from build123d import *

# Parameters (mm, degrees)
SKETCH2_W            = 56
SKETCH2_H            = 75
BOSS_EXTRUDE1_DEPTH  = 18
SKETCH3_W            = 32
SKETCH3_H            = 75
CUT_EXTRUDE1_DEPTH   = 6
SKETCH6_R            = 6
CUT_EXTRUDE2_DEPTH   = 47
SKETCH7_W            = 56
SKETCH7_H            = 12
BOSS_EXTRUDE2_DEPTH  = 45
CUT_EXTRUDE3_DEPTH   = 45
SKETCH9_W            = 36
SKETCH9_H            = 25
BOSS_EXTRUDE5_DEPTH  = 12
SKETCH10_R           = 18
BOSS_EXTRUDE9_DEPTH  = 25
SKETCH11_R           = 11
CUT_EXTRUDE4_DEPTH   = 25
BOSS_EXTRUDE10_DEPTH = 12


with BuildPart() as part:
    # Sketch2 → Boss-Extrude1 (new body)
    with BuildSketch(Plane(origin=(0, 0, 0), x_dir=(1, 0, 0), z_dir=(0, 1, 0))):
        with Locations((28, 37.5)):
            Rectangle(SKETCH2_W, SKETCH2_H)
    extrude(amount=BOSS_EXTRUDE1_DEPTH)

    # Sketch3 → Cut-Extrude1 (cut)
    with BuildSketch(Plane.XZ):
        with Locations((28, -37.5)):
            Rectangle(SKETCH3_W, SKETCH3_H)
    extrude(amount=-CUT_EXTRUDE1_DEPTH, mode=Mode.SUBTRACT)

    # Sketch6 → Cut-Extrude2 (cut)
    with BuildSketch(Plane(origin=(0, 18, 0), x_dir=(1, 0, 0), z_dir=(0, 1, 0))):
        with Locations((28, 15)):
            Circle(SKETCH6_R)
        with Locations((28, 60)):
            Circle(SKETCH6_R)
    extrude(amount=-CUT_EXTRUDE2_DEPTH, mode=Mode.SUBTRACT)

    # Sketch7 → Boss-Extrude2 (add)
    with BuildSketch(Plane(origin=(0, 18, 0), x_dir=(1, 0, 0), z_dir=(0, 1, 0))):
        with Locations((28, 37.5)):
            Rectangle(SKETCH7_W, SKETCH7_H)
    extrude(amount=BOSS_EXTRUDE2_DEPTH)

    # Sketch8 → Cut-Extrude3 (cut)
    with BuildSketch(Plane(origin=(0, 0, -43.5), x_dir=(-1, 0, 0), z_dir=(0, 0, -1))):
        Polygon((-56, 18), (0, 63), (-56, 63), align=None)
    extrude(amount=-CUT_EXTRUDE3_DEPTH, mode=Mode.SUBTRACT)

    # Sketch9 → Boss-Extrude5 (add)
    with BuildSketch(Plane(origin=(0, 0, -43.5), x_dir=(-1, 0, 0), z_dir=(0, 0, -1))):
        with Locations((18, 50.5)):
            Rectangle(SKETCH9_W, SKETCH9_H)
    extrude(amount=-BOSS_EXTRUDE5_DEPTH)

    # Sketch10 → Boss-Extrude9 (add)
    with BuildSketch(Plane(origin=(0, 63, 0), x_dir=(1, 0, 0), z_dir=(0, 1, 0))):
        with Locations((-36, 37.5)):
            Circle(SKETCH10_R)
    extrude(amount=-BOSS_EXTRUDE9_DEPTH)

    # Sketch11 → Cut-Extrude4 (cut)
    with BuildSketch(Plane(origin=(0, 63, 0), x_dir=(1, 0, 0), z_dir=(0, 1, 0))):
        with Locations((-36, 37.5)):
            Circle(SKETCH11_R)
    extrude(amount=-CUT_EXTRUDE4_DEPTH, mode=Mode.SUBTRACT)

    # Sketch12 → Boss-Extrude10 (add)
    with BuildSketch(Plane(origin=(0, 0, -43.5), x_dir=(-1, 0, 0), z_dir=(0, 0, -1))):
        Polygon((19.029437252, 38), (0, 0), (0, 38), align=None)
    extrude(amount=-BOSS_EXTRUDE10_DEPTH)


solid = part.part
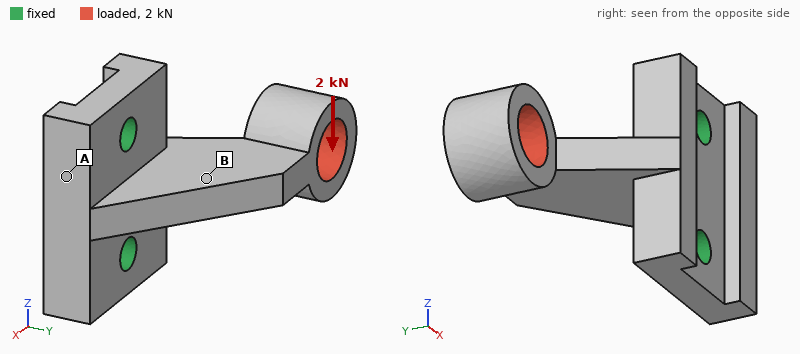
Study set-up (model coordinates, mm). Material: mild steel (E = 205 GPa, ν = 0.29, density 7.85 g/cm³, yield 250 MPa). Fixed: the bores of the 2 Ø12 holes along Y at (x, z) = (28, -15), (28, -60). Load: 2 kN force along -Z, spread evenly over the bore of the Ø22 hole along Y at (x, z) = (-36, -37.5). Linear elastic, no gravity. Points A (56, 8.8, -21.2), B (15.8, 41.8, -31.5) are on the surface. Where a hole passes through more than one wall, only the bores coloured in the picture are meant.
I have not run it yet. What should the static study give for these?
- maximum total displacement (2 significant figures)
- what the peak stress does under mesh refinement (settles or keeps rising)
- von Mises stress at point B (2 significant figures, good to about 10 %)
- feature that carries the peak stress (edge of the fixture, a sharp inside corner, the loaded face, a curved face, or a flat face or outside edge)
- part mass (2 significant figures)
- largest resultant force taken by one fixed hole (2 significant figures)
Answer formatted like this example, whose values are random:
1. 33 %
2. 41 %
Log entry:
1. 0.23 mm
2. keeps rising
3. 70 MPa
4. a sharp inside corner
5. 780 g
6. 3.3 kN
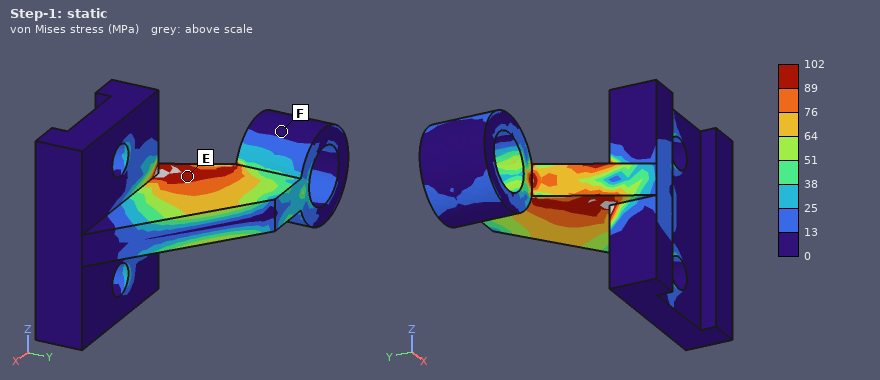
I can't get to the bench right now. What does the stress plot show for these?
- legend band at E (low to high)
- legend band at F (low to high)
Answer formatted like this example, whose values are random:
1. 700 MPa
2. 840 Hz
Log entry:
1. 89 to 102 MPa
2. 0 to 13 MPa
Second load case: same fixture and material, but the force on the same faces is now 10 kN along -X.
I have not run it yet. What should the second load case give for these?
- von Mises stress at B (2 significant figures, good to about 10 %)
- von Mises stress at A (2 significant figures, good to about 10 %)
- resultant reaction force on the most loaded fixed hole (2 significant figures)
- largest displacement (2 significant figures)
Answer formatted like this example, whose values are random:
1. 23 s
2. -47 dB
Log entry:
1. 56 MPa
2. 32 MPa
3. 5.1 kN
4. 0.16 mm
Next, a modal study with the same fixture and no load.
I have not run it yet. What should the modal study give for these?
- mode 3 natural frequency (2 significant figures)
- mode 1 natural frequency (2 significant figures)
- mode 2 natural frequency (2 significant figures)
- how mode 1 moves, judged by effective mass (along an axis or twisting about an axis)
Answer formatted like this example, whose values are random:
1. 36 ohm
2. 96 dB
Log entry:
1. 4000 Hz
2. 1500 Hz
3. 2400 Hz
4. along Z
